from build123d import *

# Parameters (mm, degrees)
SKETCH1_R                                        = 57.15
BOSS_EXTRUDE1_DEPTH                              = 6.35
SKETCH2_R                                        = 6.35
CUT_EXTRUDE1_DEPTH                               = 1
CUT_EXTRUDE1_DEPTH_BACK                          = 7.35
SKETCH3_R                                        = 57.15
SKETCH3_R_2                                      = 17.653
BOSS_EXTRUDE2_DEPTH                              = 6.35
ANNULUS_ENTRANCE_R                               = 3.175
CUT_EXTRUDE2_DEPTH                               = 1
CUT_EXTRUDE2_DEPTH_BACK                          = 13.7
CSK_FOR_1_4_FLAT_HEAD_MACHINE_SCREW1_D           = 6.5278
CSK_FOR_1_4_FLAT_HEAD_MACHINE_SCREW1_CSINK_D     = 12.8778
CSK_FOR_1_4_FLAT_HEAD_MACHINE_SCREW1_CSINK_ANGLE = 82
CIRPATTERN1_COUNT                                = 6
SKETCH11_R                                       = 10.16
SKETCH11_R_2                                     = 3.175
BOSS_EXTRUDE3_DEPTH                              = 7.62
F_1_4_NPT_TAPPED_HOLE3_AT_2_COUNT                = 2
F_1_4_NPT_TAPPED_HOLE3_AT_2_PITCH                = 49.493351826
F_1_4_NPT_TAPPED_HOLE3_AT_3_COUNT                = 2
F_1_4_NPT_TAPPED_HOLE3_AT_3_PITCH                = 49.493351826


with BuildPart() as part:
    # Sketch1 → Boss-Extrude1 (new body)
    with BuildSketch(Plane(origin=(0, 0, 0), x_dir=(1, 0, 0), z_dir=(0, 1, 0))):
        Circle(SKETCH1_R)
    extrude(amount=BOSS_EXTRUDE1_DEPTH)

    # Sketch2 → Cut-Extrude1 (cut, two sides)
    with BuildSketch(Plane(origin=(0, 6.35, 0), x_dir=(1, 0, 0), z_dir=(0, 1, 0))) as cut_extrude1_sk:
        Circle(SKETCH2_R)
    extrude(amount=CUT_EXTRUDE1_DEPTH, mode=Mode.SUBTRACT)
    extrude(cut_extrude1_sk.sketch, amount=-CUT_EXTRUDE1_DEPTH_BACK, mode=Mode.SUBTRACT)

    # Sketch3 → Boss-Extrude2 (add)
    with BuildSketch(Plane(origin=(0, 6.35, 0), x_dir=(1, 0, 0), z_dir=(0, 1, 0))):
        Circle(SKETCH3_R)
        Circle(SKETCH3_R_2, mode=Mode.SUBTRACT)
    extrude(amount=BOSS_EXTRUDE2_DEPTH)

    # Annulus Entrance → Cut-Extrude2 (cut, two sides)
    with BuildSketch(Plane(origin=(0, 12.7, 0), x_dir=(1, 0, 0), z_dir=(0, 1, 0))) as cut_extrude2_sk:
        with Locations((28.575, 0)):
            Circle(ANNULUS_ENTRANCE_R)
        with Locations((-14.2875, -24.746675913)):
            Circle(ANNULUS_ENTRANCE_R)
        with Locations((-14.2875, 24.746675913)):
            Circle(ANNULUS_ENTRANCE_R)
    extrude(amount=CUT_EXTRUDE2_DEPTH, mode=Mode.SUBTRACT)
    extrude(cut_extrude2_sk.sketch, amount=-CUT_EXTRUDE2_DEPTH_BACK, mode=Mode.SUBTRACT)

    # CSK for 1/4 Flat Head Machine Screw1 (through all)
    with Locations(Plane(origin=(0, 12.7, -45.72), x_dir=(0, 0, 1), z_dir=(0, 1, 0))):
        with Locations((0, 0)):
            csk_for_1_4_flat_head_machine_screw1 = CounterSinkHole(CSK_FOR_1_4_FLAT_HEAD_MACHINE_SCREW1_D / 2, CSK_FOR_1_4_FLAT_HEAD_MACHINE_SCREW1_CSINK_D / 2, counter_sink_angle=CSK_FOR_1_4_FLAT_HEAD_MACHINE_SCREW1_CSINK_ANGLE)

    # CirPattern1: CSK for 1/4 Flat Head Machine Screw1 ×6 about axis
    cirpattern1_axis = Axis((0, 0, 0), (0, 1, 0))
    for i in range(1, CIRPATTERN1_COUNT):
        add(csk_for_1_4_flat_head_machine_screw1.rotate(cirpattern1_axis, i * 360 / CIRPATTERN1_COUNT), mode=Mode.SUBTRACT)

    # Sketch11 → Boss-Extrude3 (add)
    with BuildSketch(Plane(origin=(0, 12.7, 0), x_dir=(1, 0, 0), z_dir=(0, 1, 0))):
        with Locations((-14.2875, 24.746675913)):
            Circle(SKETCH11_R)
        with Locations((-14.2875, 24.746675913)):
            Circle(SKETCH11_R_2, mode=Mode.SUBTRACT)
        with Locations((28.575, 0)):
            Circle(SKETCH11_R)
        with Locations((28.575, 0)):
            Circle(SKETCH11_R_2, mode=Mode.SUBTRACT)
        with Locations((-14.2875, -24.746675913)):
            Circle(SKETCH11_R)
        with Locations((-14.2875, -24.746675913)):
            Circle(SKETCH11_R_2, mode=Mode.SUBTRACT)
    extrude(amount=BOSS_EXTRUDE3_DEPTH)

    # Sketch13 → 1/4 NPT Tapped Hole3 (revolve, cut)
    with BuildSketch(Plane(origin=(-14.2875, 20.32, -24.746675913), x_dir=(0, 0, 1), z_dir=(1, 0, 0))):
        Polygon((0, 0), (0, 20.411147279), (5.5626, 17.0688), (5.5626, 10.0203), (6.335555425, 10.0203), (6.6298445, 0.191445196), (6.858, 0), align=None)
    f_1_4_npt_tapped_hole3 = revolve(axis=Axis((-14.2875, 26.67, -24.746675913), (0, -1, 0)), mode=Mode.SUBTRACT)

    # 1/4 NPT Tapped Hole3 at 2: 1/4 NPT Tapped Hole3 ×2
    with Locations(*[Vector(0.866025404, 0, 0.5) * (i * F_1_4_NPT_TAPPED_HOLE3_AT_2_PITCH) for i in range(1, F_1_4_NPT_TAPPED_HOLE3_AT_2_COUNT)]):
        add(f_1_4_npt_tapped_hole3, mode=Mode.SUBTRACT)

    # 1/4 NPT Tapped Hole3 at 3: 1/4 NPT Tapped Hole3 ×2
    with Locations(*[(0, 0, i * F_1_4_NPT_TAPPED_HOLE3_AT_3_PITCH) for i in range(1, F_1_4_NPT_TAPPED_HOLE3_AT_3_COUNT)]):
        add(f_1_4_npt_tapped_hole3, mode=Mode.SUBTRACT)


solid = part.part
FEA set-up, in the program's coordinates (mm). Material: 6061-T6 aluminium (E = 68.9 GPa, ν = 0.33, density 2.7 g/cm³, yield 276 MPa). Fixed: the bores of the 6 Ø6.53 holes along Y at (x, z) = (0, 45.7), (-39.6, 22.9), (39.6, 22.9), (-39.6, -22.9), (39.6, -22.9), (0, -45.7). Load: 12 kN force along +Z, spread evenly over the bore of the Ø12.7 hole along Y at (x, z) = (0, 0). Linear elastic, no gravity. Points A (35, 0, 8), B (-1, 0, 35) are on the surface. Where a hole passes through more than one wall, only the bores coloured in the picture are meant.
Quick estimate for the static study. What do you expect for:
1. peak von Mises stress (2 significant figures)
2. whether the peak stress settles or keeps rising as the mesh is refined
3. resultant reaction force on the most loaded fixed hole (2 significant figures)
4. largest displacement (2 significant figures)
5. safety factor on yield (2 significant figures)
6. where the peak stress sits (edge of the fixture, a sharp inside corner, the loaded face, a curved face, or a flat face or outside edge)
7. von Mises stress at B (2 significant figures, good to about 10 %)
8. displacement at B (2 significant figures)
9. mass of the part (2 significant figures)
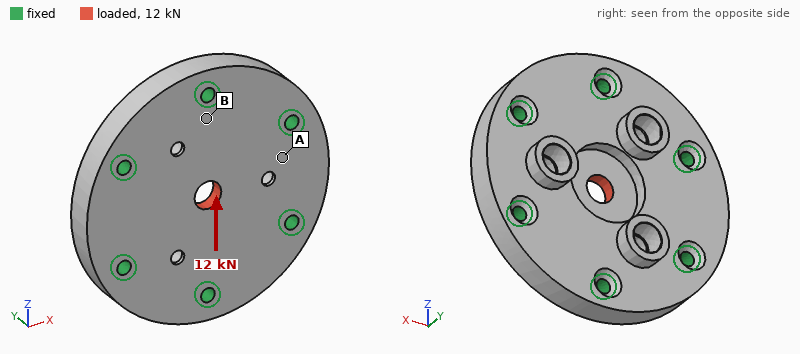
83 MPa
settles
3.1 kN
14 µm
3.3
the loaded face
20 MPa
2.2 µm
330 g
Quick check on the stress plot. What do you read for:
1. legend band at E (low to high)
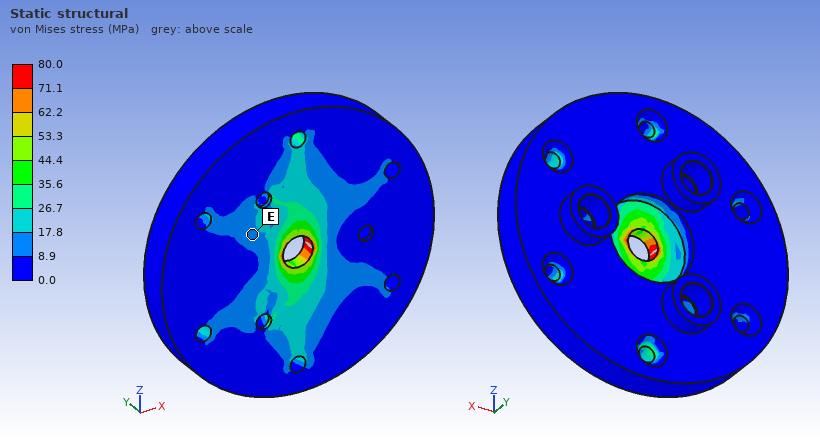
8.9 to 17.8 MPa
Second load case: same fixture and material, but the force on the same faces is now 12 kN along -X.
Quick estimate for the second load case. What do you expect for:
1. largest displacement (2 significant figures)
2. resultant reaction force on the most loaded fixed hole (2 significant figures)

14 µm
2.8 kN
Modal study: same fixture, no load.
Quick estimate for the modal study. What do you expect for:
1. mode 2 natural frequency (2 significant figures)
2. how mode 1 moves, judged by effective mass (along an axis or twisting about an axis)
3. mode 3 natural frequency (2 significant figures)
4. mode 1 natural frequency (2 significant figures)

16 kHz
along Y
16 kHz
9600 Hz
